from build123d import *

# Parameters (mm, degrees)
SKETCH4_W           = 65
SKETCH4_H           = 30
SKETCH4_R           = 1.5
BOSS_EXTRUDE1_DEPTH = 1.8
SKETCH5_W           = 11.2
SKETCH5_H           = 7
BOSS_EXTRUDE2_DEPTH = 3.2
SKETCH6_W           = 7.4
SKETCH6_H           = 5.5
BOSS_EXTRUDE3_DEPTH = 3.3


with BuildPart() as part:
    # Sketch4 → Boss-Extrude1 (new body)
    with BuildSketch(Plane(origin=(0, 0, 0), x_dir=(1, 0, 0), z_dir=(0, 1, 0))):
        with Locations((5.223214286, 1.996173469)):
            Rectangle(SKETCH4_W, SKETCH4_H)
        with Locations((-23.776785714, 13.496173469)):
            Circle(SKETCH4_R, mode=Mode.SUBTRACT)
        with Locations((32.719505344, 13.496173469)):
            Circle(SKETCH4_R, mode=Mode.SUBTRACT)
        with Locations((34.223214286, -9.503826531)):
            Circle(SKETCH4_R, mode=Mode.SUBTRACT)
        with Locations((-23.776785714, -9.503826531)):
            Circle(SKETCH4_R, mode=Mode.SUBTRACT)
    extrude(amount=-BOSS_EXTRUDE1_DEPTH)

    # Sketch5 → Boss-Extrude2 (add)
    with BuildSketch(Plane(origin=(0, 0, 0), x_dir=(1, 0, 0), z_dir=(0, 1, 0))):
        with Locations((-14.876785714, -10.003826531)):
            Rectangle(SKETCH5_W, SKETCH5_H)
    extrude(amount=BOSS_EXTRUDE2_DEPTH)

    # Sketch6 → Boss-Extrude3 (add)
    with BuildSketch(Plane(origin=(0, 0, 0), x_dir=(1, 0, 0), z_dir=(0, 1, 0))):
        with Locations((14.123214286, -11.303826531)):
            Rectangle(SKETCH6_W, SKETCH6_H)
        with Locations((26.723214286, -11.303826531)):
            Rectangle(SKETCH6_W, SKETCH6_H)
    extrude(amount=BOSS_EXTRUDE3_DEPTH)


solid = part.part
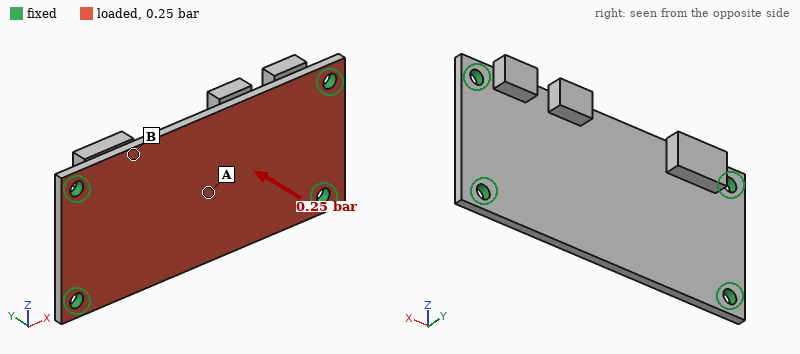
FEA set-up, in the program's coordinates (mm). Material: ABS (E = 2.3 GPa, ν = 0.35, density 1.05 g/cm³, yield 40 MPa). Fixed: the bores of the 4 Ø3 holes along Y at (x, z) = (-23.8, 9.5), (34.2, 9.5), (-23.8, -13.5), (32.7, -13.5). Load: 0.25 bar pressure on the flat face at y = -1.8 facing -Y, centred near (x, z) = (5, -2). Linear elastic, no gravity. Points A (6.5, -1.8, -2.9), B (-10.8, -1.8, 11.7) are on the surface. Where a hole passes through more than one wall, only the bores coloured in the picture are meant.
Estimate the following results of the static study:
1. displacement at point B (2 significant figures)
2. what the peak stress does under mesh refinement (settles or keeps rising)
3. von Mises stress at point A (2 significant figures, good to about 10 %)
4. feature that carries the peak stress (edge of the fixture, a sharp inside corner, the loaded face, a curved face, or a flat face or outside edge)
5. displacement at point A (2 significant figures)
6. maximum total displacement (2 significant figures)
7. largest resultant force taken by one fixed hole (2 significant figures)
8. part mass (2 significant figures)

0.29 mm
keeps rising
5.3 MPa
edge of the fixture
0.58 mm
0.63 mm
13 N
4.2 g
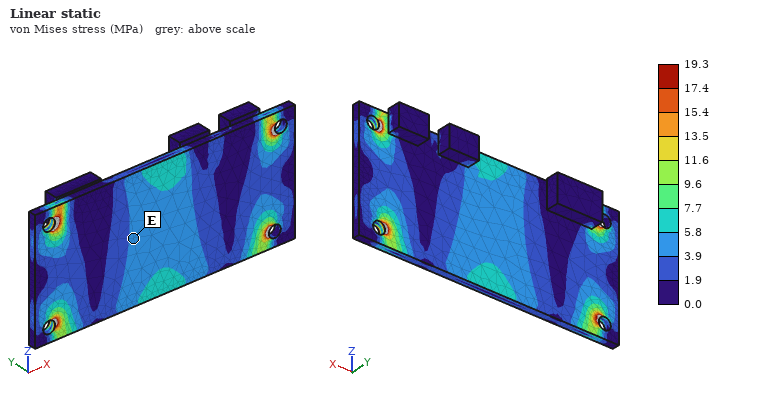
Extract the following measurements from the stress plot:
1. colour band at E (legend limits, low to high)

3.9 to 5.8 MPa
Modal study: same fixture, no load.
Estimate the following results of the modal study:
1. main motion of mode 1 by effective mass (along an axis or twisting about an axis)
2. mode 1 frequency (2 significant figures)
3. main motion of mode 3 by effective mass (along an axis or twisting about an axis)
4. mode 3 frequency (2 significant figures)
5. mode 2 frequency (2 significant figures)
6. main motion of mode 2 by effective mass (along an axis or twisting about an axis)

along Y
820 Hz
twisting about Z
2200 Hz
1400 Hz
twisting about X
